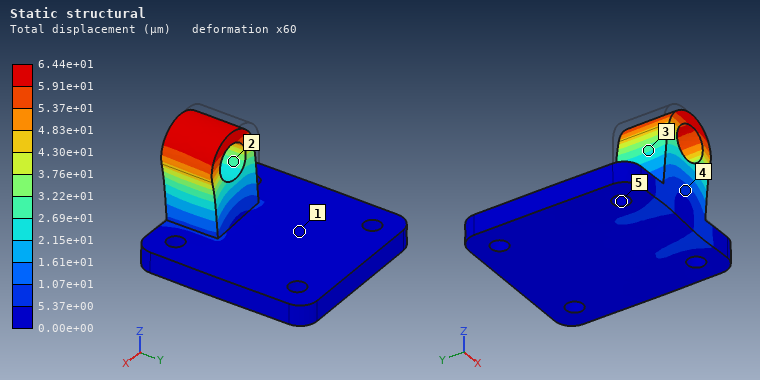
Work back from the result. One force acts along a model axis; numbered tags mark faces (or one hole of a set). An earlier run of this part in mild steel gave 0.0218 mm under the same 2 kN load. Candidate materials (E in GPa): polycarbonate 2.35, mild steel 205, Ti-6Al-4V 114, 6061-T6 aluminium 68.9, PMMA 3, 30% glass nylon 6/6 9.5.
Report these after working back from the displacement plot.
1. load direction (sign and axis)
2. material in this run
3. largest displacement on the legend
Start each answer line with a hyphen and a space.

- +X
- 6061-T6 aluminium
- 6.44e+01 µm
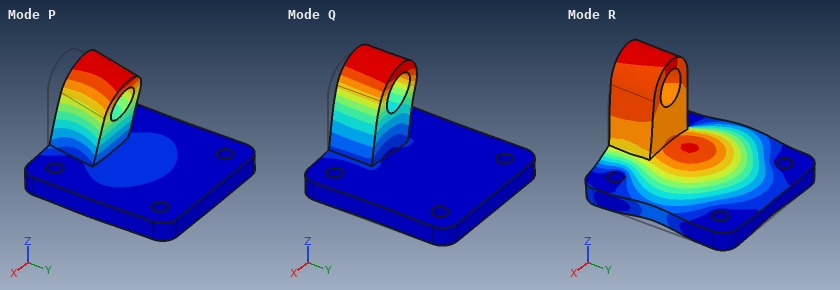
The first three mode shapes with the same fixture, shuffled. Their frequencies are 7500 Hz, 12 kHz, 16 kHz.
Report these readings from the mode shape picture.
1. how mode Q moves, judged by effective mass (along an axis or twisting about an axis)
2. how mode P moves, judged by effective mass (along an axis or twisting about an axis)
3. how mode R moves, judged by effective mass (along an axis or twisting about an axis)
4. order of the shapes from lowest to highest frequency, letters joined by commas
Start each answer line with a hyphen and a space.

- along X
- along Y
- along Z
- P, Q, R
